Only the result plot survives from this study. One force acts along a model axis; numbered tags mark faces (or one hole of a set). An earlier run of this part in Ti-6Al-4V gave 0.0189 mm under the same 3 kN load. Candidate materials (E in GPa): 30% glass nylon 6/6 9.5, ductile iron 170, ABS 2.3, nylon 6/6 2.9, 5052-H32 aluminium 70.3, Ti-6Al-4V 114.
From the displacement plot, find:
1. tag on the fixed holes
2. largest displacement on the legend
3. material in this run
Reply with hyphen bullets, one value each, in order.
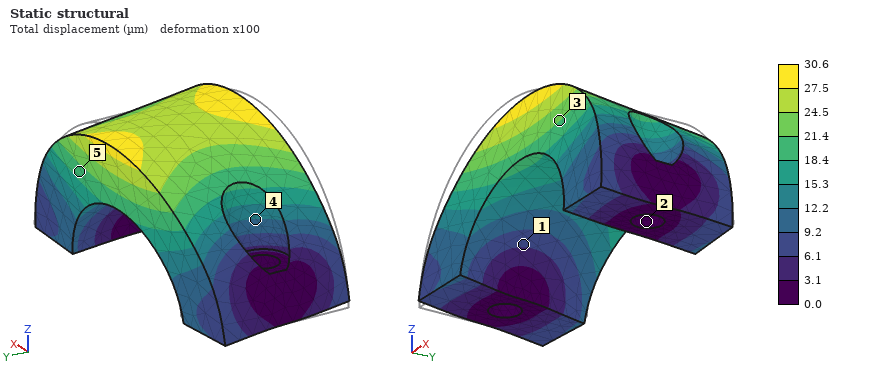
- 2
- 30.6 µm
- 5052-H32 aluminium
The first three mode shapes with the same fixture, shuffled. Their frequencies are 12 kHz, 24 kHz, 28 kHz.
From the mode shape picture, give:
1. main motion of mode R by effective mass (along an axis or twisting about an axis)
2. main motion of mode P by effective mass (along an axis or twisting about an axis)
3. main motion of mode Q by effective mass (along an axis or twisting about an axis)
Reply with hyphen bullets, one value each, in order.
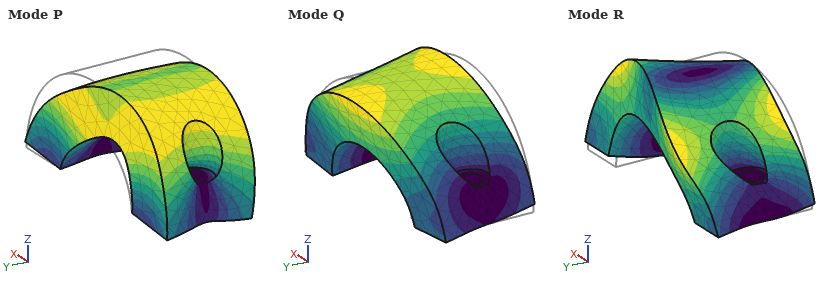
- twisting about Z
- along X
- along Y
